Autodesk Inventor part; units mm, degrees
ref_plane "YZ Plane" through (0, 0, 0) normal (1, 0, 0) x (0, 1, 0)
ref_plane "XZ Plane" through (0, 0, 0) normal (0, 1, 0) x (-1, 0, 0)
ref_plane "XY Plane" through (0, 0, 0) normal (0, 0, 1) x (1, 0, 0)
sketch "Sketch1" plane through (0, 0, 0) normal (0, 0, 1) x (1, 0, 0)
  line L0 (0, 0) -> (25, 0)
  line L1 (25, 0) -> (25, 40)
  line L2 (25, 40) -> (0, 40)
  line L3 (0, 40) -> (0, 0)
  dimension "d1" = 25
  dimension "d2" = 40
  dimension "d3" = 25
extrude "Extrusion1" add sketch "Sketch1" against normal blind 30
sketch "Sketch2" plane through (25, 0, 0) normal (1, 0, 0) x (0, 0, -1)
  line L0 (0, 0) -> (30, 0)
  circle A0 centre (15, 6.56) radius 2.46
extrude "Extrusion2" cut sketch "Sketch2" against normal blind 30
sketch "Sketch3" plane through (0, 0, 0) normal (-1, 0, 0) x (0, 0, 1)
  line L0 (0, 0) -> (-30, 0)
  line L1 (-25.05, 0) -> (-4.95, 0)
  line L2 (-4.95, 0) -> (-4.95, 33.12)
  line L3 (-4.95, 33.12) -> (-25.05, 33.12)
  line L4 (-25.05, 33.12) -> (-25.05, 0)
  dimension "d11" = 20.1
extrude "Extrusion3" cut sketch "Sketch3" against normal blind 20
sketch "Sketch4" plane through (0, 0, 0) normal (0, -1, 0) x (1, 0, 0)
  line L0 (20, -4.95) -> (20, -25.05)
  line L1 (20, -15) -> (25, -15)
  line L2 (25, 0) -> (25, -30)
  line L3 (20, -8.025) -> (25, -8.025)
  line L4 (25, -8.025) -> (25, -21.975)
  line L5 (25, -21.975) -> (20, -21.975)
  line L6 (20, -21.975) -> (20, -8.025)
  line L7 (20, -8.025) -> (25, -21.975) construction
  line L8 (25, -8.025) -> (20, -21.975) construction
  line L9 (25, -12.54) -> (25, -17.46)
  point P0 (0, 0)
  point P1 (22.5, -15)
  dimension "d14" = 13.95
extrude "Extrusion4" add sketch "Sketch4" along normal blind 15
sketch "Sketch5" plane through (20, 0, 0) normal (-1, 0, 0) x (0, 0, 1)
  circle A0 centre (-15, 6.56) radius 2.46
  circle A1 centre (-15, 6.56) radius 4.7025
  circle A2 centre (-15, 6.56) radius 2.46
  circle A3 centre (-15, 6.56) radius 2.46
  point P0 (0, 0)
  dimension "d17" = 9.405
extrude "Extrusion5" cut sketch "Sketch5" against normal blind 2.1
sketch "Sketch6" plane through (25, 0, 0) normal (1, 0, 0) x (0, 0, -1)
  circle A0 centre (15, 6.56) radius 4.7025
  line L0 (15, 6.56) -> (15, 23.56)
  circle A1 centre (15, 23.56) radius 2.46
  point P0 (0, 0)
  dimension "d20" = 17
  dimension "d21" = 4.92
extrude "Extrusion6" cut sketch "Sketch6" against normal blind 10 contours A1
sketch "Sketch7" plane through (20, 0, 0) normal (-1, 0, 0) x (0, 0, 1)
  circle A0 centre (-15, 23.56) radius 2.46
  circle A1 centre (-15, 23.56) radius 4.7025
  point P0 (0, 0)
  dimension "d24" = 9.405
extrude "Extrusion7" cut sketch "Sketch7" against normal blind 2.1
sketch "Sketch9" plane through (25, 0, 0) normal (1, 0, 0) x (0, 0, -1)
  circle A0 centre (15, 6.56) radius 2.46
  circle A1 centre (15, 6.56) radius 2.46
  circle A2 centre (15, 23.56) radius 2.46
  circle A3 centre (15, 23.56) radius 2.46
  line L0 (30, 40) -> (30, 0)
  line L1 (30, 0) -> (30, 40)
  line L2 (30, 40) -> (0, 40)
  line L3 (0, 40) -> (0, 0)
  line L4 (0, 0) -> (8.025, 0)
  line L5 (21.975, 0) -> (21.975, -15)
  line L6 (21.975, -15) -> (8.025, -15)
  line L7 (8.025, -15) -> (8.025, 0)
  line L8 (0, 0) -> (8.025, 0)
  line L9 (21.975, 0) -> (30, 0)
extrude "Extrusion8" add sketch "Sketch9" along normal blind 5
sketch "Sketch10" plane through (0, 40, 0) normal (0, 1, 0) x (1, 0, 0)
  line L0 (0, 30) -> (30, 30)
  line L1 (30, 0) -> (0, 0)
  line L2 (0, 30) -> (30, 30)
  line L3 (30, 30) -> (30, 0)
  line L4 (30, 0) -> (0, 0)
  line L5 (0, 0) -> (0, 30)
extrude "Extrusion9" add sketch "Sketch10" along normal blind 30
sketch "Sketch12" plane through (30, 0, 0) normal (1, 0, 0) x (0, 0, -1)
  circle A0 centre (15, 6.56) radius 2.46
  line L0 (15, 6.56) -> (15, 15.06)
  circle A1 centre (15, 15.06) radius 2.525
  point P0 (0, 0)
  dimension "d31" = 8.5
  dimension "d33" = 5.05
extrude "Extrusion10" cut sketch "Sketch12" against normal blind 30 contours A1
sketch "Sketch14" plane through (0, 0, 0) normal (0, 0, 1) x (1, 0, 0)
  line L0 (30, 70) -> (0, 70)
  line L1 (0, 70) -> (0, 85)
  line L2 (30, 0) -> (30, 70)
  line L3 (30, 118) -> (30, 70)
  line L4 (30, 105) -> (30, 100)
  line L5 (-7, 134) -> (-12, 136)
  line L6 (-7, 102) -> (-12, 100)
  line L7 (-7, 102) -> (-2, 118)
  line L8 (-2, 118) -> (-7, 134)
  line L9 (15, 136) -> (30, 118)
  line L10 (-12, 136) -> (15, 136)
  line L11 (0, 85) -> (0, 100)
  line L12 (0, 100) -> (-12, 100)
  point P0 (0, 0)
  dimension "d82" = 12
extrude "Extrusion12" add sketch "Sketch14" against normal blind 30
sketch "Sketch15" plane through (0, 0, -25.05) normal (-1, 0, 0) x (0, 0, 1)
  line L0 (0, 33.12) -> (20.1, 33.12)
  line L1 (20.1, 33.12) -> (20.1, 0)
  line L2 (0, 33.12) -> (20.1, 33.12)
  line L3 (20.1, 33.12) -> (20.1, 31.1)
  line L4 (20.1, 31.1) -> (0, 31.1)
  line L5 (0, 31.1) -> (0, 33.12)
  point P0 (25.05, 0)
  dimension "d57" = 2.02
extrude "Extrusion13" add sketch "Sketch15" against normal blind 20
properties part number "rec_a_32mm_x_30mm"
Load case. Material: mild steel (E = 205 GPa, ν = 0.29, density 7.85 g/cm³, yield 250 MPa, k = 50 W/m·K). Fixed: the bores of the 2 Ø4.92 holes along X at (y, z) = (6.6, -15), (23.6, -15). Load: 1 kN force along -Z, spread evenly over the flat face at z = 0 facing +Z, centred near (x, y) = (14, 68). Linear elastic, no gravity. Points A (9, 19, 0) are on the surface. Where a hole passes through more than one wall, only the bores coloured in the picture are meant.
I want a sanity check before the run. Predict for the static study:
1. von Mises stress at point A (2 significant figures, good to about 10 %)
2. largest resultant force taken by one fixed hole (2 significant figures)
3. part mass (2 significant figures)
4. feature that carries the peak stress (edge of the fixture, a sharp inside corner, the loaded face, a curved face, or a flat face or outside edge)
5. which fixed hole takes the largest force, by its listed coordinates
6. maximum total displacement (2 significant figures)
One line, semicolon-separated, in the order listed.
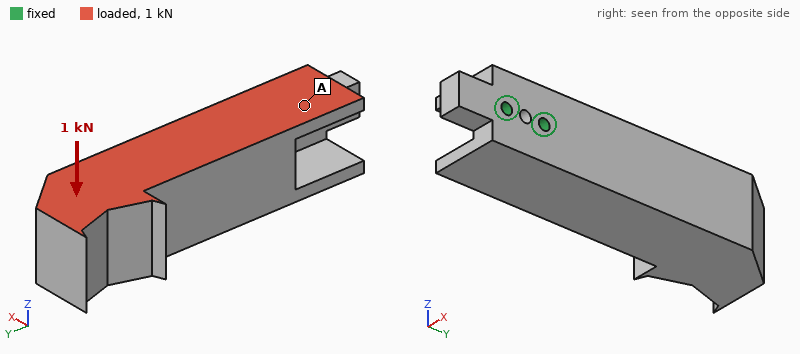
7.1 MPa; 2.9 kN; 880 g; edge of the fixture; (23.6, -15); 39 µm
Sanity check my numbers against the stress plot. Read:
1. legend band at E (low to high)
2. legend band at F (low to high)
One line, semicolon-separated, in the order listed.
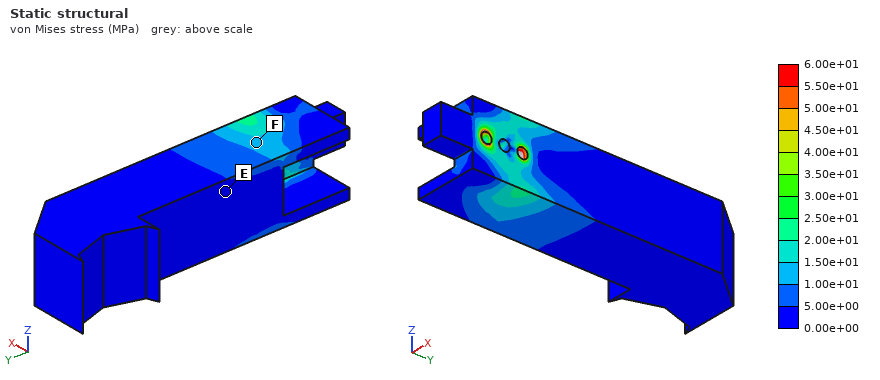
0.00e+00 to 5.00e+00 MPa; 1.00e+01 to 1.50e+01 MPa
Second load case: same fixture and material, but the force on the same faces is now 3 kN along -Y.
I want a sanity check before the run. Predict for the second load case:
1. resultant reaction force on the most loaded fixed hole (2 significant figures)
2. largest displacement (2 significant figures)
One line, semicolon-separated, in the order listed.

3.0 kN; 46 µm
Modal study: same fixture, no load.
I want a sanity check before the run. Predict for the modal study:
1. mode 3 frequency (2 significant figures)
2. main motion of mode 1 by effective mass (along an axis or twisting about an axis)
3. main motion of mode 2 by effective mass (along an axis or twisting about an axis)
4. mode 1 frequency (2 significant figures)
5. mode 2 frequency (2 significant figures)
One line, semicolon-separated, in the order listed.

3000 Hz; along X; along Z; 890 Hz; 1000 Hz
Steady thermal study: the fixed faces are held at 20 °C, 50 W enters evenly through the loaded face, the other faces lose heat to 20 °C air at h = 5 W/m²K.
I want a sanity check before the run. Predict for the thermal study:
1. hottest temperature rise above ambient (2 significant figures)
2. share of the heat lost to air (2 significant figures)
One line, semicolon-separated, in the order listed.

75 K; 7.7 %
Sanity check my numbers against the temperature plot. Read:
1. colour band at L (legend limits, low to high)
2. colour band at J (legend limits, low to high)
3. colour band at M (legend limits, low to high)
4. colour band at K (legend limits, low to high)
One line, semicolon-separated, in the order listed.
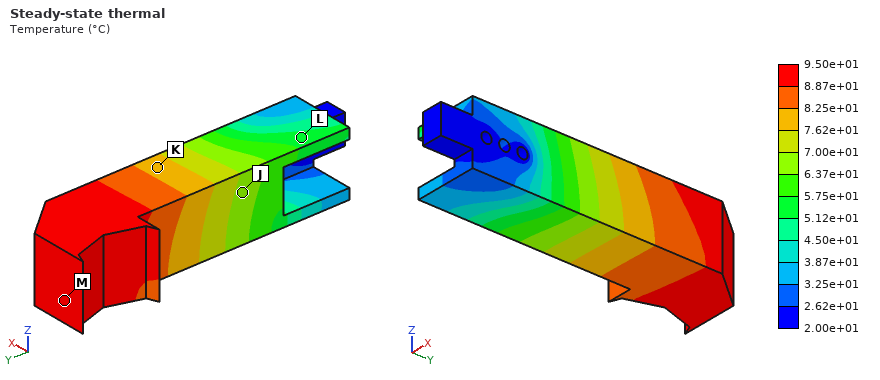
5.12e+01 to 5.75e+01 °C; 6.37e+01 to 7.00e+01 °C; 8.87e+01 to 9.50e+01 °C; 7.62e+01 to 8.25e+01 °C
